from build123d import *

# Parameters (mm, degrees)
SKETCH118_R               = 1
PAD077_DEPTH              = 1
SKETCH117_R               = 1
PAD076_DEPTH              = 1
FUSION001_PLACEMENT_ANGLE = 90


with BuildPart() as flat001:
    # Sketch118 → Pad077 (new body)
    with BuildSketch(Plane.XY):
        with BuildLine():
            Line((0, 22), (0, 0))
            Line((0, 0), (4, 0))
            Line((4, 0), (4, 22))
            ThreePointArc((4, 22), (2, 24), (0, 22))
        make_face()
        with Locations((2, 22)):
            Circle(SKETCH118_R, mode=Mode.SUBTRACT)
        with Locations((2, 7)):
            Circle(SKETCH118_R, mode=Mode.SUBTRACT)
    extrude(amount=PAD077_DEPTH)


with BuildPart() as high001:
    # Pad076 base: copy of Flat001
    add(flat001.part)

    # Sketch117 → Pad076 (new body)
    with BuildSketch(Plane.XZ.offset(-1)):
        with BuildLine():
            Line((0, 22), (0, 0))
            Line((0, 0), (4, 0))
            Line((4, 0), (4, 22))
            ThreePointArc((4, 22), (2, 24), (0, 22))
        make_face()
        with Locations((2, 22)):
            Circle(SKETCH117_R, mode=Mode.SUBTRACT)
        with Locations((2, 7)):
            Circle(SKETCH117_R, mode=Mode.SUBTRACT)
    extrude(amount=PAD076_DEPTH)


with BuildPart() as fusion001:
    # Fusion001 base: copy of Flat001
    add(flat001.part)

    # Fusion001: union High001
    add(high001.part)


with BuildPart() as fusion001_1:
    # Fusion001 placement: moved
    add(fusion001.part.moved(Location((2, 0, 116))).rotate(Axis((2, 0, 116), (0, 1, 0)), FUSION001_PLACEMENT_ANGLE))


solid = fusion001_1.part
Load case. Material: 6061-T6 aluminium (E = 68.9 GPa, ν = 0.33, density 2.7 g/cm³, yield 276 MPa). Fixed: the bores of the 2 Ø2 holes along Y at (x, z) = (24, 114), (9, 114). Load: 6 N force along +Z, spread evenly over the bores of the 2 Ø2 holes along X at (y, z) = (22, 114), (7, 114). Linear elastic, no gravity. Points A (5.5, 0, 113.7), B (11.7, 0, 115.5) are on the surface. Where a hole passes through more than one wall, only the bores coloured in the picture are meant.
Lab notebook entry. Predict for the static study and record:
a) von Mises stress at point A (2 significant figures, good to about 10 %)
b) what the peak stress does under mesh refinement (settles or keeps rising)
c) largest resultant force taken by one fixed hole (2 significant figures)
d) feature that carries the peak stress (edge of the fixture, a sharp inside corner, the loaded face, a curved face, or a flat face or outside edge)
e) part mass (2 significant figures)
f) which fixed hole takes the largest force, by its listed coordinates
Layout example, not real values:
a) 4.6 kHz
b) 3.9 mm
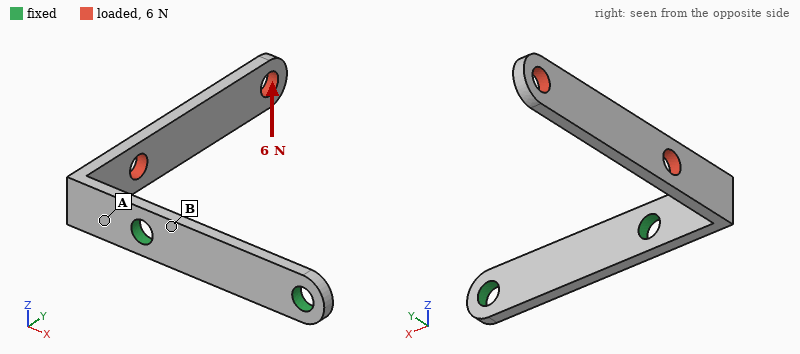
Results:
a) 110 MPa
b) keeps rising
c) 6.3 N
d) edge of the fixture
e) 0.46 g
f) (9, 114)
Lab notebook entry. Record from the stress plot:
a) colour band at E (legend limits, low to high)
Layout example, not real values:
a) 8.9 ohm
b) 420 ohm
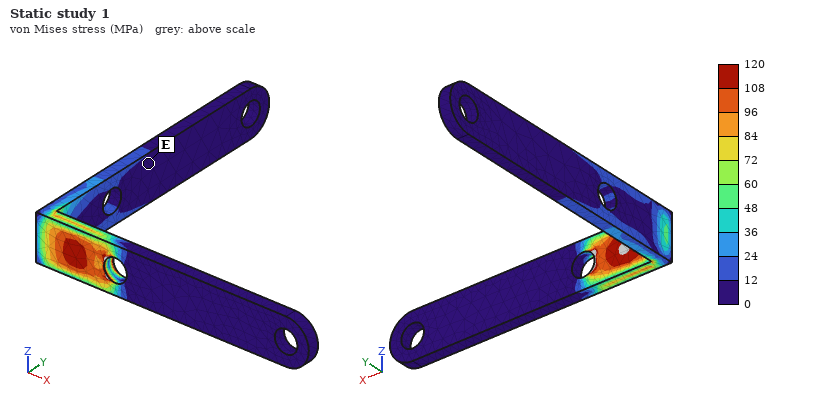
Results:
a) 0 to 12 MPa
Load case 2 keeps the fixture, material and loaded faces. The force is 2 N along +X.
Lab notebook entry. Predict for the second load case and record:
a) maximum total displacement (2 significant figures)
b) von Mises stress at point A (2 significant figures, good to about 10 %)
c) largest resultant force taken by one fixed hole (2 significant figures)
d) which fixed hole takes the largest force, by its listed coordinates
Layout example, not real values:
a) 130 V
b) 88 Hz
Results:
a) 0.36 mm
b) 39 MPa
c) 2.0 N
d) (9, 114)
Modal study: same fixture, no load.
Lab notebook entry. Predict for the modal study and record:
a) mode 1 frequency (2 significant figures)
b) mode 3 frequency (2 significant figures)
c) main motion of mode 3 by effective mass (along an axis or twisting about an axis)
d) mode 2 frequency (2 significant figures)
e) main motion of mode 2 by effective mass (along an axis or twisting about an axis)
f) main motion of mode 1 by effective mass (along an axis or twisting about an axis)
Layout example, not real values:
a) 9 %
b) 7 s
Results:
a) 1100 Hz
b) 6300 Hz
c) along Y
d) 1900 Hz
e) along Z
f) along X
